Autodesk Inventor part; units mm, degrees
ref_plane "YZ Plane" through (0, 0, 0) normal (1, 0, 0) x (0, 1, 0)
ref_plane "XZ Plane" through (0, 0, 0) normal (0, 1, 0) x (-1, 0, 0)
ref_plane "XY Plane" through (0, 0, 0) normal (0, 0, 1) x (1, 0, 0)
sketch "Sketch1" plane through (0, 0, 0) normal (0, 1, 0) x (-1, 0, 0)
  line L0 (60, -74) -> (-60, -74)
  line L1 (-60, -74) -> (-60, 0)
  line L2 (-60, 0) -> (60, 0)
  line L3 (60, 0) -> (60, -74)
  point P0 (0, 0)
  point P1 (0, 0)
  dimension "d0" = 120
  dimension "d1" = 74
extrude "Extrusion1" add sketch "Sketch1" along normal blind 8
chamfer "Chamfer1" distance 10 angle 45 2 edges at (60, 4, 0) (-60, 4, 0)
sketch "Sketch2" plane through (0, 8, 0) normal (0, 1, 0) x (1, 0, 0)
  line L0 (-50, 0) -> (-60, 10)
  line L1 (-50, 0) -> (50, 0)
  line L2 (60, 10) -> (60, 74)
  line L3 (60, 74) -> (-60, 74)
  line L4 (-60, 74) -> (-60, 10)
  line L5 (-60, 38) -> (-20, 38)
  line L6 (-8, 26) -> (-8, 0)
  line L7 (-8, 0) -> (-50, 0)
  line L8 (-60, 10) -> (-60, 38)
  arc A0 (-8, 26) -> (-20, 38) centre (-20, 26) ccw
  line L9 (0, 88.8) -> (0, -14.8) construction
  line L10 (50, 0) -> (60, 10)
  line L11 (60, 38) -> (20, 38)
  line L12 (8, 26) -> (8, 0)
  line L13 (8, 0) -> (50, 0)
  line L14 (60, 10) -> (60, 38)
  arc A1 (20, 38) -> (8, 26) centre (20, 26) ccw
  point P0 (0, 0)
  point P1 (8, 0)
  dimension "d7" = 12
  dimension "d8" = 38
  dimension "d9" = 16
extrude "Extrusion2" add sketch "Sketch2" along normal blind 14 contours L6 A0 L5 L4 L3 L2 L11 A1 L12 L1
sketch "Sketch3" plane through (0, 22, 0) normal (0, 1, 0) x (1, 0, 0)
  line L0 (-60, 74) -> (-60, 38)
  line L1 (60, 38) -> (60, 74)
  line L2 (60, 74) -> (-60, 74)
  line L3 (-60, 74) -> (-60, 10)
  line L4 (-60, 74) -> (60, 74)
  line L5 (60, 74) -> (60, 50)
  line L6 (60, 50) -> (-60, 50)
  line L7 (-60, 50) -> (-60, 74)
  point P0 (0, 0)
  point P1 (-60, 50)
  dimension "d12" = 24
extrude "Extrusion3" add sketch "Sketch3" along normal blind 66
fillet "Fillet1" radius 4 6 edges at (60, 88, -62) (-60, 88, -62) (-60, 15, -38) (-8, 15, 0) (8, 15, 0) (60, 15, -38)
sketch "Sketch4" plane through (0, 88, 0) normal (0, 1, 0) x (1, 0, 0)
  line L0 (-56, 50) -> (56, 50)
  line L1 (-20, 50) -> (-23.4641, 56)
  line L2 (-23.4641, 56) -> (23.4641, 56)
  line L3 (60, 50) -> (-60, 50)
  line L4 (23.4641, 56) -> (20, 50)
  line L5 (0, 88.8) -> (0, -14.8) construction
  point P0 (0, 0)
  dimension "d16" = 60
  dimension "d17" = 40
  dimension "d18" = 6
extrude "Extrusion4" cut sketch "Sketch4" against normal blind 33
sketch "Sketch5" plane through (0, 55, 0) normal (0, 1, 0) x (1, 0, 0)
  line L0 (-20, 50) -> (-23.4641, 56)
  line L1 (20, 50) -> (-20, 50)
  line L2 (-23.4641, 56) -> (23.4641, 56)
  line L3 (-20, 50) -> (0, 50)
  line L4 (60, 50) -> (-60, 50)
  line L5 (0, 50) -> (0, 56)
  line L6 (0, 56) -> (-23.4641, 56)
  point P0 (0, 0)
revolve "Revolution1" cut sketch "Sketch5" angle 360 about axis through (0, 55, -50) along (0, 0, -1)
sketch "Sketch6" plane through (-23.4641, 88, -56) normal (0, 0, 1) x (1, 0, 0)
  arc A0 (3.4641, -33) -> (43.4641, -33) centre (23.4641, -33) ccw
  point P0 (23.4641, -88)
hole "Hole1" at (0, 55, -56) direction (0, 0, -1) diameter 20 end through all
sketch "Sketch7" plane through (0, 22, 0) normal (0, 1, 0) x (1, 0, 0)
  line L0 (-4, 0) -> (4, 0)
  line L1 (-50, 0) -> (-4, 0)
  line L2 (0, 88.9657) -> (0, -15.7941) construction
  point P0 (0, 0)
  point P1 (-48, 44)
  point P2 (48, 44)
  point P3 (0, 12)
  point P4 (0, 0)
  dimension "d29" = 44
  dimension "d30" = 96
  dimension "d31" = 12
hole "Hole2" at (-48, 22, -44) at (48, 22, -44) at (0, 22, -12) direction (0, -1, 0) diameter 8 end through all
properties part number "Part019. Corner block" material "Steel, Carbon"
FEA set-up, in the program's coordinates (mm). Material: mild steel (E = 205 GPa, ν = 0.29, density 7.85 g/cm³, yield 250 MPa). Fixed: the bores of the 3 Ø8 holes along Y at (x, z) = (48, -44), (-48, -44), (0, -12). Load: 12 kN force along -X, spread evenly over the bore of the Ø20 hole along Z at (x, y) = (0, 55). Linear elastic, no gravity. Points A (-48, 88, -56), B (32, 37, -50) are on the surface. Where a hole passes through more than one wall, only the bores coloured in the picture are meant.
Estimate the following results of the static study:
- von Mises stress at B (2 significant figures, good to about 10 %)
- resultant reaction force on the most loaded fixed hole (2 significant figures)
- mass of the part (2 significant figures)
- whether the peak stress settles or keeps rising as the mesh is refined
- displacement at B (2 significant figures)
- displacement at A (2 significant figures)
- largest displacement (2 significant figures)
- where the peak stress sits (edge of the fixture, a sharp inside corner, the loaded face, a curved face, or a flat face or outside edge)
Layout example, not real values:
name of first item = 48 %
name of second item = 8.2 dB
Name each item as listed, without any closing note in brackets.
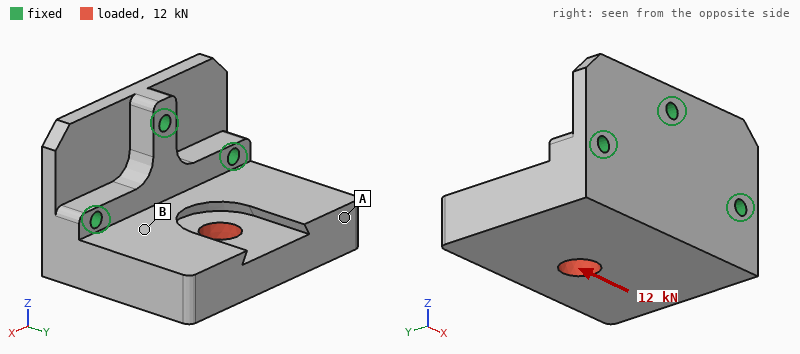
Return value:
von Mises stress at B = 10 MPa
resultant reaction force on the most loaded fixed hole = 8.0 kN
mass of the part = 2.4 kg
whether the peak stress settles or keeps rising as the mesh is refined = keeps rising
displacement at B = 4.0 µm
displacement at A = 9.7 µm
largest displacement = 10 µm
where the peak stress sits = edge of the fixture
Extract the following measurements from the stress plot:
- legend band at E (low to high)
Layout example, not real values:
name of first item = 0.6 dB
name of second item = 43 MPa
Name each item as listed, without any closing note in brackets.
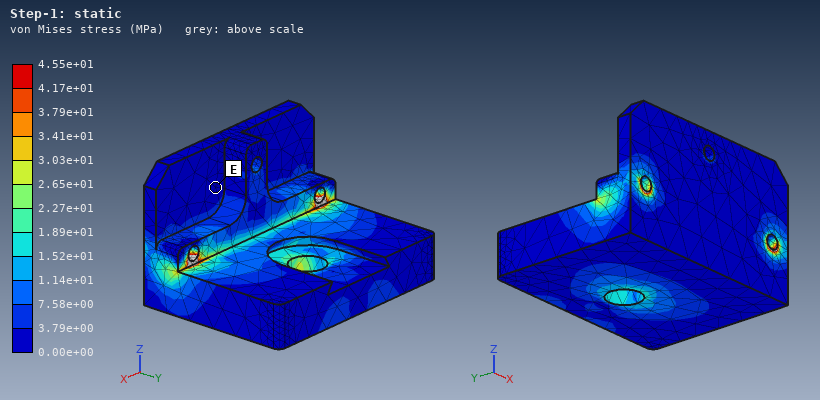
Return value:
legend band at E = 0.00e+00 to 3.79e+00 MPa
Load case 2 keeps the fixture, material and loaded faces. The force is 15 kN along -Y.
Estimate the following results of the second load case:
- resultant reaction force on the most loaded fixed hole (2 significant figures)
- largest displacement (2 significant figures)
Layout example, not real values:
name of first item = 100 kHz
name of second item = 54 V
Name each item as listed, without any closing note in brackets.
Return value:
resultant reaction force on the most loaded fixed hole = 7.9 kN
largest displacement = 32 µm
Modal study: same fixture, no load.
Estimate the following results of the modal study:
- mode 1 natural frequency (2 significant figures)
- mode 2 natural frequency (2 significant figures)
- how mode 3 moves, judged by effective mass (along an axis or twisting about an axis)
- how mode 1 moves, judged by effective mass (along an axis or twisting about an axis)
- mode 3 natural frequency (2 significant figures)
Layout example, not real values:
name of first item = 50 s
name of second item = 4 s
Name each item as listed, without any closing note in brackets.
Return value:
mode 1 natural frequency = 2100 Hz
mode 2 natural frequency = 4000 Hz
how mode 3 moves, judged by effective mass = along X
how mode 1 moves, judged by effective mass = along Z
mode 3 natural frequency = 6000 Hz
